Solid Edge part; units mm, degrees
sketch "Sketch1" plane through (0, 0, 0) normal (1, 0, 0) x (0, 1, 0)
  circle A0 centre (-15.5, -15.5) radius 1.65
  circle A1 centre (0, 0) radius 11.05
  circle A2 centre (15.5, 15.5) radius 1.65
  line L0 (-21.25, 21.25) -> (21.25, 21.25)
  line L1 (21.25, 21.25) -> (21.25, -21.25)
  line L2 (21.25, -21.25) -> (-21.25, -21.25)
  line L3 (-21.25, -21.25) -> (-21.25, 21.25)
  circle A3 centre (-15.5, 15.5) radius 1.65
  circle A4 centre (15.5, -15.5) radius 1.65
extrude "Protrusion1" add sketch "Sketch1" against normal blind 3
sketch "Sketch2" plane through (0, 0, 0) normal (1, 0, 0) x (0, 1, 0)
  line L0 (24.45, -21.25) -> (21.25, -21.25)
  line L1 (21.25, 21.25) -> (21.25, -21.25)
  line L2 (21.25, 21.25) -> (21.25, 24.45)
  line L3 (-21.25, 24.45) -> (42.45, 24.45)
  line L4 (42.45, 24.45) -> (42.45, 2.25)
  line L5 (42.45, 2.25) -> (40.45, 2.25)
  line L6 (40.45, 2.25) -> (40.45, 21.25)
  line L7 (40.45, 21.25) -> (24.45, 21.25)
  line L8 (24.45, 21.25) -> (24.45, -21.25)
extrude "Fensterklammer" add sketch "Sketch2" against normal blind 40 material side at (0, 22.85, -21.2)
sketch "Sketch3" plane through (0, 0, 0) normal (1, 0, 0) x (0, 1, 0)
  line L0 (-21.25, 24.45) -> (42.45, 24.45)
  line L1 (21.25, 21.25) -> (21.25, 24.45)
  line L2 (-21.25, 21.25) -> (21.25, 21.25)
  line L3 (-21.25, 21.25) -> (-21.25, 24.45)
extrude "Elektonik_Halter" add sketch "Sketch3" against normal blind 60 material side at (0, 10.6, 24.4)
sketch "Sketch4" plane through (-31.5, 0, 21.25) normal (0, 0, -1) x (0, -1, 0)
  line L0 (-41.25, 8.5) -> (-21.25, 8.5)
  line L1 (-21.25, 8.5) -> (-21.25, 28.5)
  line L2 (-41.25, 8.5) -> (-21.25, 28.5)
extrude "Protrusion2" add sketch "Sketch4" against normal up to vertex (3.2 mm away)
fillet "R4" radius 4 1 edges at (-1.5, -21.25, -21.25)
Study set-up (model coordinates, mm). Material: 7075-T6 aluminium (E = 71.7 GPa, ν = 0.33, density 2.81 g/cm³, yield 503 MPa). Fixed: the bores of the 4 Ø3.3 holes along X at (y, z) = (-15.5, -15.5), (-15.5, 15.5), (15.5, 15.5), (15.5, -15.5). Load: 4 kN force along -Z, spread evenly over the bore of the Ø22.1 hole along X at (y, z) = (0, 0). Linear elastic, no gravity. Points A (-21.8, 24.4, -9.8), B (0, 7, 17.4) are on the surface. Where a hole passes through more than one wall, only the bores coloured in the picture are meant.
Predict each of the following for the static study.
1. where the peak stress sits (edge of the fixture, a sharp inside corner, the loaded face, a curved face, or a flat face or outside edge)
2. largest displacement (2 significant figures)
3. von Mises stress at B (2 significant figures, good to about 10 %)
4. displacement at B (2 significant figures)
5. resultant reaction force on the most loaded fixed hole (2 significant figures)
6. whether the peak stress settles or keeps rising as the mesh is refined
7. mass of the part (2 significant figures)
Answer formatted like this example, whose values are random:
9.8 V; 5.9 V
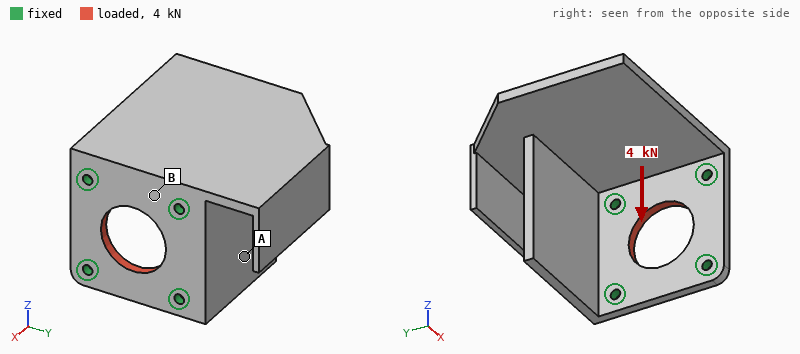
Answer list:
edge of the fixture; 12 µm; 19 MPa; 5.1 µm; 1.0 kN; keeps rising; 64 g
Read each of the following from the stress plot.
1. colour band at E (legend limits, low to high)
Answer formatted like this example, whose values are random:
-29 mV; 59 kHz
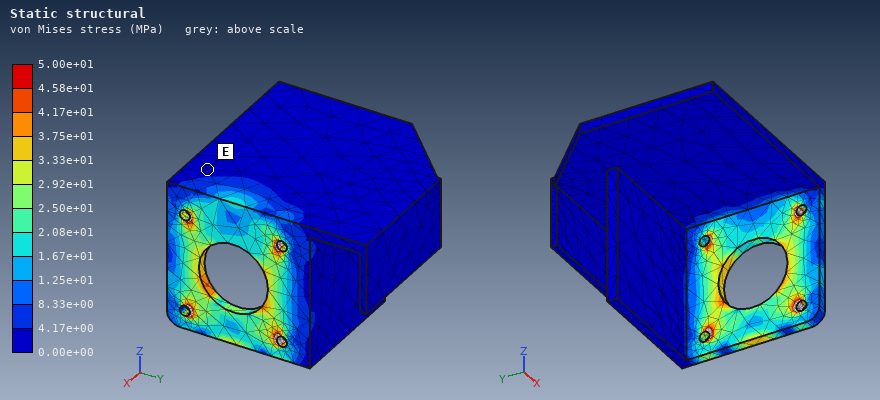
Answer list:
0.00e+00 to 4.17e+00 MPa
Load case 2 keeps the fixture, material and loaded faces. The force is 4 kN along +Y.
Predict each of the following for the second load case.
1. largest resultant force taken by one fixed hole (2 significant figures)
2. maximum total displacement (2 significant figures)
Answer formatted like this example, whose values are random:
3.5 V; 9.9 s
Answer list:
1.0 kN; 12 µm
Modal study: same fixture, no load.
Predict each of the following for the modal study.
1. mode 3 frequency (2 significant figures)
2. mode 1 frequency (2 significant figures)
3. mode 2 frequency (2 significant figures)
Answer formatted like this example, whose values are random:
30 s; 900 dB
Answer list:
2700 Hz; 1300 Hz; 2200 Hz
